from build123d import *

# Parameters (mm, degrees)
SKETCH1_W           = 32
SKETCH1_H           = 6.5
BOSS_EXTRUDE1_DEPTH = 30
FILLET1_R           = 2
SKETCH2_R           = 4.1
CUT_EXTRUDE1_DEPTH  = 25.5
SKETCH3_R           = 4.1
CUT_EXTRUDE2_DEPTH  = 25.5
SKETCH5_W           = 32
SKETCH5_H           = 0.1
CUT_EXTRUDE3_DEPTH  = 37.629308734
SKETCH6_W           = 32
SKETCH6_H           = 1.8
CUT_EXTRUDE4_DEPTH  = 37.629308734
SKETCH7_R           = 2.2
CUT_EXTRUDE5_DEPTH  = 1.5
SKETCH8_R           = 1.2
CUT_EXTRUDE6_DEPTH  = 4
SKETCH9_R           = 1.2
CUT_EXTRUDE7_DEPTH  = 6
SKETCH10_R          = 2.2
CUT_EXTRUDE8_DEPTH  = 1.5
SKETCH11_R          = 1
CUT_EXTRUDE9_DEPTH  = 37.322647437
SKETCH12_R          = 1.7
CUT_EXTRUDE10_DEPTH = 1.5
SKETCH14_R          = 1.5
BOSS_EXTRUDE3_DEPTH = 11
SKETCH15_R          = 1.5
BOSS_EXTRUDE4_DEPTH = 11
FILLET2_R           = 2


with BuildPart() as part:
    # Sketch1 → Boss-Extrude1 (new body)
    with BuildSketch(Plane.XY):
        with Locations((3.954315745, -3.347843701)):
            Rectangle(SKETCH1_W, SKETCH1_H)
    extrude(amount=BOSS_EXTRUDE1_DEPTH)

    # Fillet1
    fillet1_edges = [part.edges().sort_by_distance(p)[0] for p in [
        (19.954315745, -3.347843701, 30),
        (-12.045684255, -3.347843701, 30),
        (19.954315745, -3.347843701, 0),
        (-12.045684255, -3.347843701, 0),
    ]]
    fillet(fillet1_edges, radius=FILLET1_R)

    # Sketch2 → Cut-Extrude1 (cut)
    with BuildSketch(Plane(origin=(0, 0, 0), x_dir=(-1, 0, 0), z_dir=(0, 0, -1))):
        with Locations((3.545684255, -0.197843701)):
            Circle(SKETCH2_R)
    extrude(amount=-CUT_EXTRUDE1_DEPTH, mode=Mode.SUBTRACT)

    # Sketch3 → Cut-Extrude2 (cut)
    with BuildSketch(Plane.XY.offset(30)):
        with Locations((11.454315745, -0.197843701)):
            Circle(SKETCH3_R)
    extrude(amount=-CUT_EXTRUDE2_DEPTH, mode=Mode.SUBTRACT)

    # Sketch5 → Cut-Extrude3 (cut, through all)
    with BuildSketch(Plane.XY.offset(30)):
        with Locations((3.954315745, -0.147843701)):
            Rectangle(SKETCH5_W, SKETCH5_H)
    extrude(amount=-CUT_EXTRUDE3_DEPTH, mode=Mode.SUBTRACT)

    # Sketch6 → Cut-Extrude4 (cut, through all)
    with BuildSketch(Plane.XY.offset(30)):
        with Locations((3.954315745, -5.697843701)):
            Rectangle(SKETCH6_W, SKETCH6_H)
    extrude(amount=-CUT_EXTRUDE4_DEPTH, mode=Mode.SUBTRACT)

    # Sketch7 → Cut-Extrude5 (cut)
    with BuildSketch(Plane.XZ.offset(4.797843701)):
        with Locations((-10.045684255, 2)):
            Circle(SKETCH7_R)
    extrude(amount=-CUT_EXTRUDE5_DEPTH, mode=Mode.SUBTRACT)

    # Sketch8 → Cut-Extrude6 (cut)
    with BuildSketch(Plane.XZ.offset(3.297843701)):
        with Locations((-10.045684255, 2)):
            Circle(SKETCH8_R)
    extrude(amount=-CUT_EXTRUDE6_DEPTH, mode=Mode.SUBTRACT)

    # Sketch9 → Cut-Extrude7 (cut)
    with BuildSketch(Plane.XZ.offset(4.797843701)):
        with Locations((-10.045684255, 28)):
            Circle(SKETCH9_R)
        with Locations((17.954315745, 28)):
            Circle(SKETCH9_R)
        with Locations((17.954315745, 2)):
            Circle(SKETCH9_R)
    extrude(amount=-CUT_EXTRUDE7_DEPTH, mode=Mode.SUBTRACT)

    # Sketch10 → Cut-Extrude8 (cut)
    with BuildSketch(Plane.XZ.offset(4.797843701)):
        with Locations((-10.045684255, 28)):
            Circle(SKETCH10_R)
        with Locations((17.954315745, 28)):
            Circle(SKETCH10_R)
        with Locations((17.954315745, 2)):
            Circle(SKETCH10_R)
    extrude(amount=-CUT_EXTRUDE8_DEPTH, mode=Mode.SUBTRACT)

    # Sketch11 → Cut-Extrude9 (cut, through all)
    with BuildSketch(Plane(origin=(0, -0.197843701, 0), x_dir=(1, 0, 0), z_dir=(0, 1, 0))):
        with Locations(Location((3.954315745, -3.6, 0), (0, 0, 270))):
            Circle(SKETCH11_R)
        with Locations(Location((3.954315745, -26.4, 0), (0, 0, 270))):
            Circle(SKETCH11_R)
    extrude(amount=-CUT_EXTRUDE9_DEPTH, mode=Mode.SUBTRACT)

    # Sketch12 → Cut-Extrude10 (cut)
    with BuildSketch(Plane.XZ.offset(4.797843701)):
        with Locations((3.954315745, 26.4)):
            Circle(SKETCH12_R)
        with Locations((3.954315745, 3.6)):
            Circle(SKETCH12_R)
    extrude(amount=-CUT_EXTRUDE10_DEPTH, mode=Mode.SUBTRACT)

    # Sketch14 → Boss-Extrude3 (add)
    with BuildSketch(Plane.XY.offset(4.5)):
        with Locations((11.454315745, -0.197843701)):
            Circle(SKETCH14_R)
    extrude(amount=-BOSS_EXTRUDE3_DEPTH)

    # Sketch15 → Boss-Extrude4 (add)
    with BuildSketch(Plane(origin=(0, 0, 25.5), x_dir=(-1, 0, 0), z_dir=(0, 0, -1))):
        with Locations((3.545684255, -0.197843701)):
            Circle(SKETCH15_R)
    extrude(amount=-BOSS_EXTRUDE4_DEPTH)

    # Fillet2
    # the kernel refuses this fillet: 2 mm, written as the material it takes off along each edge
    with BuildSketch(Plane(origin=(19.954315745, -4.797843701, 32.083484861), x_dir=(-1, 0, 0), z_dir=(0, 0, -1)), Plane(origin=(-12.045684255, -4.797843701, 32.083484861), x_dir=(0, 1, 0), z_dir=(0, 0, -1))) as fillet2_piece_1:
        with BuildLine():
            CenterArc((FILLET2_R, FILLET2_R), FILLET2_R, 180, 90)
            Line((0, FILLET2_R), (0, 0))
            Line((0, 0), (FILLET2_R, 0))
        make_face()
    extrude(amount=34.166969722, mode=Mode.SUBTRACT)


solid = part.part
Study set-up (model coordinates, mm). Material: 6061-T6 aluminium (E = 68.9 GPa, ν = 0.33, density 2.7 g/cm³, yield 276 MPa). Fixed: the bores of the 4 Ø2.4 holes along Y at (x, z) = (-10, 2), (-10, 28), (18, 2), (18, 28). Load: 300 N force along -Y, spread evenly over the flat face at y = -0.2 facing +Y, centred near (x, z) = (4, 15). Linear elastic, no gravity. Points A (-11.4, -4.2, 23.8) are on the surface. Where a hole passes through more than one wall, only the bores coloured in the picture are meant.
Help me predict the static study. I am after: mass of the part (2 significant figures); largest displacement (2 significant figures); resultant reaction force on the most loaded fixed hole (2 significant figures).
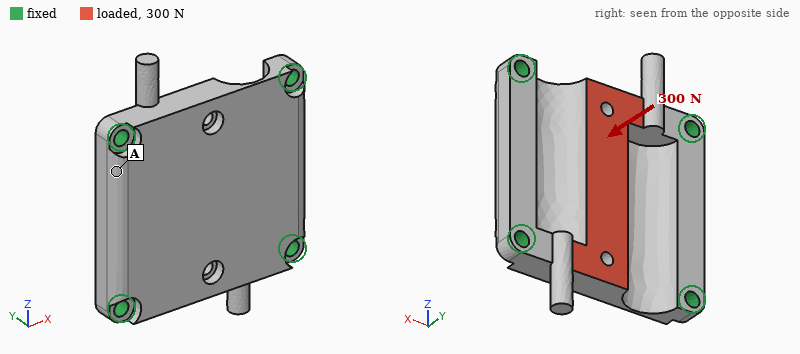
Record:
8.0 g
16 µm
140 N
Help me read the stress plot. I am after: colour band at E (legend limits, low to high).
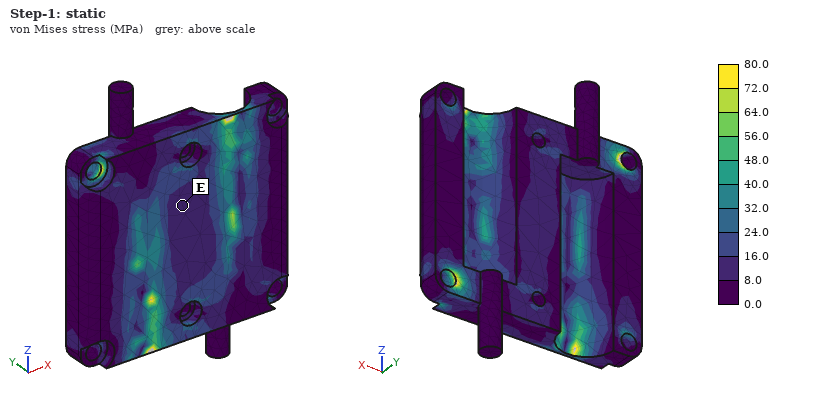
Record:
8.0 to 16.0 MPa
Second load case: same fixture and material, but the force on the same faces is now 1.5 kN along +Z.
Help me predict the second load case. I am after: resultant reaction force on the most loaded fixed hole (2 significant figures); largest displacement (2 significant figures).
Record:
450 N
49 µm
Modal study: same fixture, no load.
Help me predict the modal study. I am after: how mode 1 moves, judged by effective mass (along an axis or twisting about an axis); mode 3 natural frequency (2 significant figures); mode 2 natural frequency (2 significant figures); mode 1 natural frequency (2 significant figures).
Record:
along Y
24 kHz
15 kHz
12 kHz
